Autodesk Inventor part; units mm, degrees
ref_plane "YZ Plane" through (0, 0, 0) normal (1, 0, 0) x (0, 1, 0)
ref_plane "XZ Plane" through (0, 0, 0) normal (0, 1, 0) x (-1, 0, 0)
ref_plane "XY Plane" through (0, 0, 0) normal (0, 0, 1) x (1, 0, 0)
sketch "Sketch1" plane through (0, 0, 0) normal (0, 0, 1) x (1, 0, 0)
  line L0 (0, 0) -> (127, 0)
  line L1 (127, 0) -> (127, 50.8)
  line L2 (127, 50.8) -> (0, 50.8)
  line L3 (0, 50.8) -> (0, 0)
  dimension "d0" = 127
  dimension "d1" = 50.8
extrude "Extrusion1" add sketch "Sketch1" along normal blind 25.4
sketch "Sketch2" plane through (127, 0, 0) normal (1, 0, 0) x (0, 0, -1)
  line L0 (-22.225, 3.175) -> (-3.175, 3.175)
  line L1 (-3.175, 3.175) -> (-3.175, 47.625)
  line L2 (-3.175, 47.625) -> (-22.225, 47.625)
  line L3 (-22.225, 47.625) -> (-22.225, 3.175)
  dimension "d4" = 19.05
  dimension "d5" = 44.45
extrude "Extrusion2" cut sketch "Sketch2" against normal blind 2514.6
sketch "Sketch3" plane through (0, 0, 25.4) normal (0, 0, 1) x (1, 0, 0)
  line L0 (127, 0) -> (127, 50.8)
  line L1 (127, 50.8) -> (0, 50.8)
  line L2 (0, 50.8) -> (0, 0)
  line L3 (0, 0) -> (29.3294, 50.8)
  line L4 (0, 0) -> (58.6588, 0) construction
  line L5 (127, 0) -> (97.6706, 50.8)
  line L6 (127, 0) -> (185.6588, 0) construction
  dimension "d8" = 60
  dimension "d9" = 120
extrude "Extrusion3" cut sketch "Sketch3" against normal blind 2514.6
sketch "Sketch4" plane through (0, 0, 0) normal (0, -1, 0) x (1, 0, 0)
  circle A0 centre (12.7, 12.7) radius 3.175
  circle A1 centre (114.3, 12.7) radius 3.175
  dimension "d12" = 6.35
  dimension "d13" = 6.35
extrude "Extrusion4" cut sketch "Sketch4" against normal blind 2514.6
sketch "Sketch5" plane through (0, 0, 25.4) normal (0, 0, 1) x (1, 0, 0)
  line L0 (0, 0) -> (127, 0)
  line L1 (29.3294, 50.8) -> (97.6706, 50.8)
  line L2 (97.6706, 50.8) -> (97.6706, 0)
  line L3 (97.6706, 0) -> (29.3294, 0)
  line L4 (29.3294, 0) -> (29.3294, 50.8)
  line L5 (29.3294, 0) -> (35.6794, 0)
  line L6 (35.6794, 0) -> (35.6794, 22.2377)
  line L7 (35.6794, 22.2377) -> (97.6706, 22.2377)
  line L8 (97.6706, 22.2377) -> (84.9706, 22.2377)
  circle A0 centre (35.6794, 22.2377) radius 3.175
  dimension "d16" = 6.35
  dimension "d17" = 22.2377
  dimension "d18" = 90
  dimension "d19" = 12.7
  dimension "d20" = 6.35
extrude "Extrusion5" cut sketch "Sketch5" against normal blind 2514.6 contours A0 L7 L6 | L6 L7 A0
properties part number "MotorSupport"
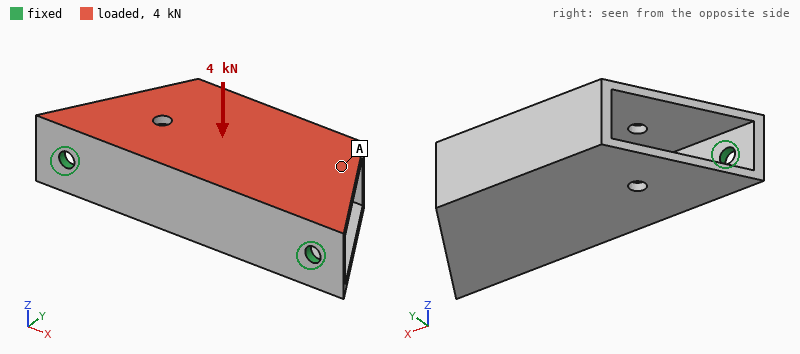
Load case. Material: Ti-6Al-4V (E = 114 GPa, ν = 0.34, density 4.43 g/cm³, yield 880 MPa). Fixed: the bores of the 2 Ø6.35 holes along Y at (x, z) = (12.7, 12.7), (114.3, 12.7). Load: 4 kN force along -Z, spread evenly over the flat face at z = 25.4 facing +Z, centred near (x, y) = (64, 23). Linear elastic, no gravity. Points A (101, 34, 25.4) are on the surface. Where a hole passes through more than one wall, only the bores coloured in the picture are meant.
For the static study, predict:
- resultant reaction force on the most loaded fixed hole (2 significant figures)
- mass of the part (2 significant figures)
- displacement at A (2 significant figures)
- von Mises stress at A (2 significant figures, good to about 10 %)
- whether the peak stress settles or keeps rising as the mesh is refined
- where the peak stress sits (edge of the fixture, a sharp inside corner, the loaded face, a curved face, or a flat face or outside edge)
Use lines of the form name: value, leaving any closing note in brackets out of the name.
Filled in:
resultant reaction force on the most loaded fixed hole: 2.0 kN
mass of the part: 190 g
displacement at A: 0.73 mm
von Mises stress at A: 61 MPa
whether the peak stress settles or keeps rising as the mesh is refined: keeps rising
where the peak stress sits: edge of the fixture
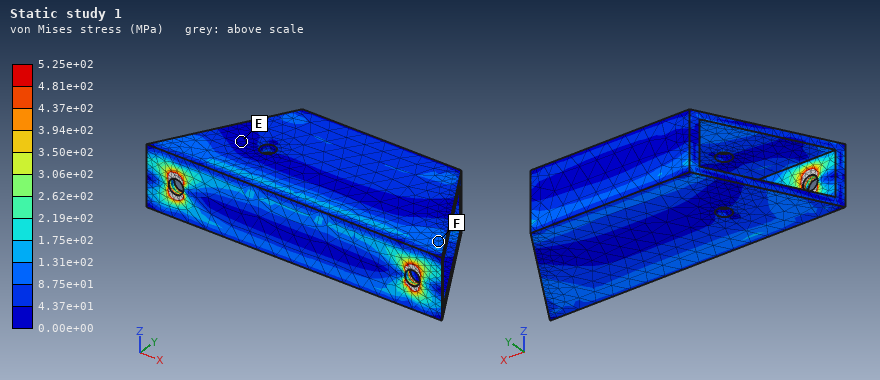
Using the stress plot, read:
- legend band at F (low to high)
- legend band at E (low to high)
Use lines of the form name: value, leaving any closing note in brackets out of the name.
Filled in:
legend band at F: 8.75e+01 to 1.31e+02 MPa
legend band at E: 0.00e+00 to 4.37e+01 MPa
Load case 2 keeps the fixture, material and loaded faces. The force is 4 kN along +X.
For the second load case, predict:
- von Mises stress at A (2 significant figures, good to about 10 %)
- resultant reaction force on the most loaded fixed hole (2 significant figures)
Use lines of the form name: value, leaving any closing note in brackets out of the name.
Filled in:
von Mises stress at A: 14 MPa
resultant reaction force on the most loaded fixed hole: 2.2 kN
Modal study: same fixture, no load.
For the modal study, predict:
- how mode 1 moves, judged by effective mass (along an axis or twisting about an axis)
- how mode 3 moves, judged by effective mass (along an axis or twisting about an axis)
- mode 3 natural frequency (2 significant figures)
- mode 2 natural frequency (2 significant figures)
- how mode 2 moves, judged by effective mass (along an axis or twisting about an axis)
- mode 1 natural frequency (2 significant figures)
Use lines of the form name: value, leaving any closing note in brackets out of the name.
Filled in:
how mode 1 moves, judged by effective mass: along Z
how mode 3 moves, judged by effective mass: twisting about Y
mode 3 natural frequency: 4000 Hz
mode 2 natural frequency: 3800 Hz
how mode 2 moves, judged by effective mass: along Y
mode 1 natural frequency: 870 Hz
